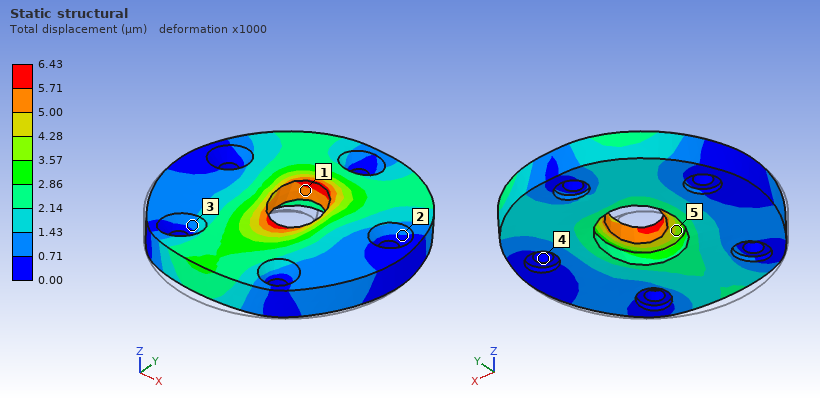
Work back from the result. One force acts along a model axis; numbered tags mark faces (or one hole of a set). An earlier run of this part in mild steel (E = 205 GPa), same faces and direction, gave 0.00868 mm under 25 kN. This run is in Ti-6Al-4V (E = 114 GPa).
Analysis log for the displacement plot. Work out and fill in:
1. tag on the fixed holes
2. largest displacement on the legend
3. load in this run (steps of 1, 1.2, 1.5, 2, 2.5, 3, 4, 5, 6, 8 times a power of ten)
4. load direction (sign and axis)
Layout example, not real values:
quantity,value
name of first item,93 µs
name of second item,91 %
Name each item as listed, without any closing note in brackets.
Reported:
quantity,value
tag on the fixed holes,4
largest displacement on the legend,6.43 µm
load in this run,10 kN
load direction,+Y
